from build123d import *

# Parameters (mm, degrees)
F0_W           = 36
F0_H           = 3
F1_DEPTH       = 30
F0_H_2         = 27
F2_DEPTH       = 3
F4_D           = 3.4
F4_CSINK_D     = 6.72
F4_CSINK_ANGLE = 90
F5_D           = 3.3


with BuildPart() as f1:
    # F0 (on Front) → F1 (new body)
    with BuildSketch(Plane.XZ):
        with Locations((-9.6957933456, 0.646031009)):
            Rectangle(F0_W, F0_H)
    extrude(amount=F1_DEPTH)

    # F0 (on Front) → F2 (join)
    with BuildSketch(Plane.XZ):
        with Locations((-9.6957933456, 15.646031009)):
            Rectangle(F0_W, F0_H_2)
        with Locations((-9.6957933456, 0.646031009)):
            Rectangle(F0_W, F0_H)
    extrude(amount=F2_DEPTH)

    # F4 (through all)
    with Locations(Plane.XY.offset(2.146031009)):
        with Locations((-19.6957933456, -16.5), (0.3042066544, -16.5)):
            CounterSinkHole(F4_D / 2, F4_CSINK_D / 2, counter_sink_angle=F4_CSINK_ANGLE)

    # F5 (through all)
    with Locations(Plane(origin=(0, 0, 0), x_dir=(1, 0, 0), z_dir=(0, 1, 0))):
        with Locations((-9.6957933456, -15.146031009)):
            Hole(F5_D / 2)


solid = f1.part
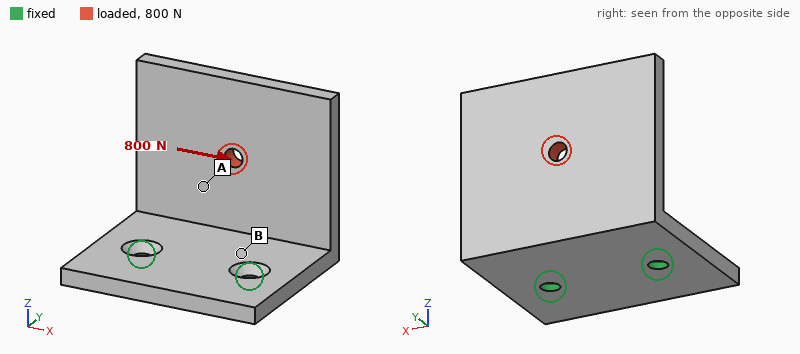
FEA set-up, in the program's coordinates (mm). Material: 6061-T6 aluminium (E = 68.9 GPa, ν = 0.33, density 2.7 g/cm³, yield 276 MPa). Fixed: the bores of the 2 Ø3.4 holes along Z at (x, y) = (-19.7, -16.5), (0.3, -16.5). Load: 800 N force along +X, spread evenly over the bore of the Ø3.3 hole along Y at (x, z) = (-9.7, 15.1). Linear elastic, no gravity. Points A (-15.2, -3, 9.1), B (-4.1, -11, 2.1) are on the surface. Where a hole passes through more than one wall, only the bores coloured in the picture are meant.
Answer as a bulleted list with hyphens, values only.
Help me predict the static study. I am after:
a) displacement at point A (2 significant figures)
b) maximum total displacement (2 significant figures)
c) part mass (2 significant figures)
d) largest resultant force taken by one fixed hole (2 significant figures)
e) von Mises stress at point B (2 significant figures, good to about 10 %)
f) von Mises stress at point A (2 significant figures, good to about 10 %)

- 0.11 mm
- 0.35 mm
- 16 g
- 890 N
- 120 MPa
- 50 MPa
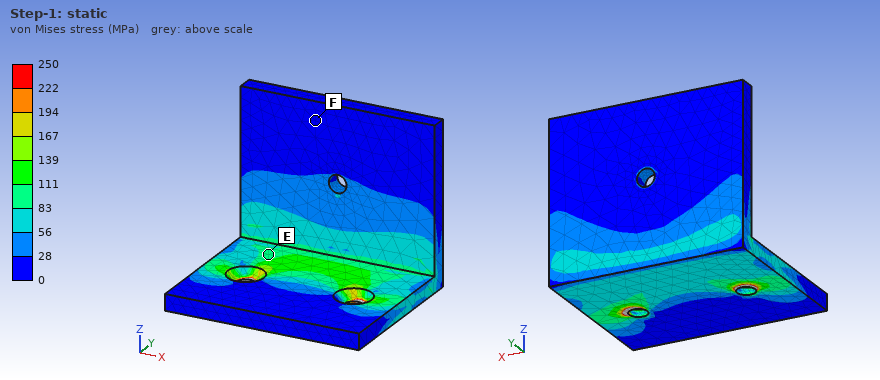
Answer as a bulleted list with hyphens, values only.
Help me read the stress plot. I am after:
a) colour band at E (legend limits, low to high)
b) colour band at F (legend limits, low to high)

- 83 to 111 MPa
- 0 to 28 MPa
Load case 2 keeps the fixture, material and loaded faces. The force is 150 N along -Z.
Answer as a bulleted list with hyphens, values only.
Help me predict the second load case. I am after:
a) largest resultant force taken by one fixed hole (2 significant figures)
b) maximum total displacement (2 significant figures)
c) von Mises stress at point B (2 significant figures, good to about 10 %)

- 78 N
- 0.15 mm
- 27 MPa
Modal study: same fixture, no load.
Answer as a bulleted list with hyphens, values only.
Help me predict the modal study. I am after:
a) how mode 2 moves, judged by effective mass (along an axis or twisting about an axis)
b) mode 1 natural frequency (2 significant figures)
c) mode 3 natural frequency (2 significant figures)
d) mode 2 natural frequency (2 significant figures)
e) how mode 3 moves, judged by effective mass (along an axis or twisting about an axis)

- along X
- 1400 Hz
- 4600 Hz
- 2900 Hz
- along Z
